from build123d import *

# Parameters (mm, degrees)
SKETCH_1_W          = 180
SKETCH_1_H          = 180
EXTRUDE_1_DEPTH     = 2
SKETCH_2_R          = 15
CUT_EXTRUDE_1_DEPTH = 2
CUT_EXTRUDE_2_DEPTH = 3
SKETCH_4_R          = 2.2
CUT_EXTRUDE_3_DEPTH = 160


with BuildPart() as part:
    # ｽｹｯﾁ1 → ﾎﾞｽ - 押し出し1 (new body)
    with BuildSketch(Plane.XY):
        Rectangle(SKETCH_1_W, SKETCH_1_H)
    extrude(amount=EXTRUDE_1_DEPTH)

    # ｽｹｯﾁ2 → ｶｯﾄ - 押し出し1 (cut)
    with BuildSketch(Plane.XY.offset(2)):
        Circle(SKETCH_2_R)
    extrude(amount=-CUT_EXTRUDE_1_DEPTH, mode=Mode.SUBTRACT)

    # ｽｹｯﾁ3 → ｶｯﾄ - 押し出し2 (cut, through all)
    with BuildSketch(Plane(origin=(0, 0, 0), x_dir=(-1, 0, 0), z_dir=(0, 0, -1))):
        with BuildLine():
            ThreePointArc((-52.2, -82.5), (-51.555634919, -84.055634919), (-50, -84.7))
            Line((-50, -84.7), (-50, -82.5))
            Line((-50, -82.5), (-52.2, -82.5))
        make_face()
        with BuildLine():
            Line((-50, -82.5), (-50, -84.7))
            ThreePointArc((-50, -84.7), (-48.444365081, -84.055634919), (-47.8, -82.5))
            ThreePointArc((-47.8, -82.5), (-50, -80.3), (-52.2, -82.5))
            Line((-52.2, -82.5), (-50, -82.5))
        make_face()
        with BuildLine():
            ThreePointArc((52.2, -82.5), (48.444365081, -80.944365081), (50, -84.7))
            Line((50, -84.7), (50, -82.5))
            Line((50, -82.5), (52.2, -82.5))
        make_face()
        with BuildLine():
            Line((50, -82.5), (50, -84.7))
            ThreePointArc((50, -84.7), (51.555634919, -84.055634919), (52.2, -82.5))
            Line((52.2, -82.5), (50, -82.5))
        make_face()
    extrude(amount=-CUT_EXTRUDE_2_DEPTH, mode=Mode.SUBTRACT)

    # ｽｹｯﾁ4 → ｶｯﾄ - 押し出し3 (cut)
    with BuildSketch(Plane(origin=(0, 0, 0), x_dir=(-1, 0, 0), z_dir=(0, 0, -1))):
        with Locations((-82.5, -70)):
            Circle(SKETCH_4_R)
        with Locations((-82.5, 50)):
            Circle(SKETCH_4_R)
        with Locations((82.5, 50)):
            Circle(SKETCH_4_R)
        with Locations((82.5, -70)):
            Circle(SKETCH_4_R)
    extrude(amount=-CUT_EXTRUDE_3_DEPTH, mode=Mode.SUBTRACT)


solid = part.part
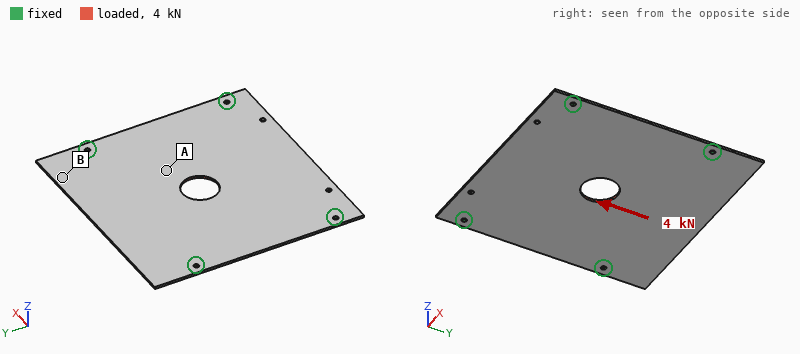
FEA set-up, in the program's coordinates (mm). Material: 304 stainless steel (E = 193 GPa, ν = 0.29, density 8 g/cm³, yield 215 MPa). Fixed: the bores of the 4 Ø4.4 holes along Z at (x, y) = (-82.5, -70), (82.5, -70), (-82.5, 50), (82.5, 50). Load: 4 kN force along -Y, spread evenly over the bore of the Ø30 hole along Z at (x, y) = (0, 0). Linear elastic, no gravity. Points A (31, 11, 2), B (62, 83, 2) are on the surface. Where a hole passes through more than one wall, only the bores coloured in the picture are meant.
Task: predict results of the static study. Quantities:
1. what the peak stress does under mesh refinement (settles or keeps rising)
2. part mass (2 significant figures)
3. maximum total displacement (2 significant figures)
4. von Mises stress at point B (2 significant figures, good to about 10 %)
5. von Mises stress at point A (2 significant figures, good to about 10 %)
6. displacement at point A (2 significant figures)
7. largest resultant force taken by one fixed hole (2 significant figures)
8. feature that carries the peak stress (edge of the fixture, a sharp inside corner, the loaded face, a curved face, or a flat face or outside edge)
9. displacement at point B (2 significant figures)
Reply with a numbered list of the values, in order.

1. keeps rising
2. 510 g
3. 11 µm
4. 5.5 MPa
5. 14 MPa
6. 7.7 µm
7. 1.1 kN
8. edge of the fixture
9. 5.0 µm
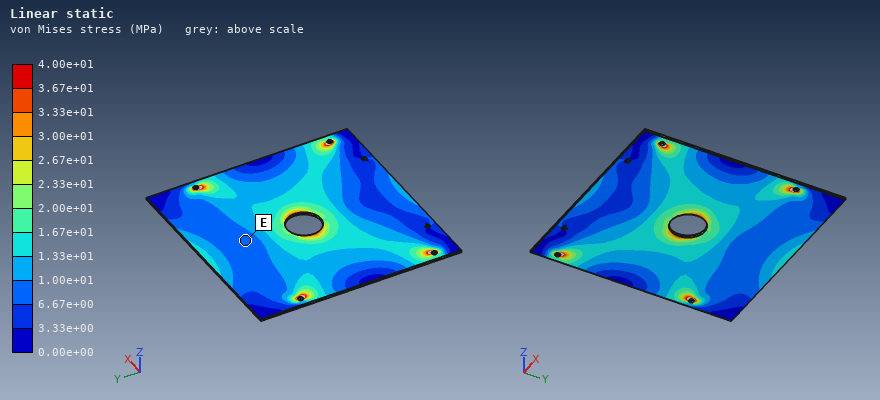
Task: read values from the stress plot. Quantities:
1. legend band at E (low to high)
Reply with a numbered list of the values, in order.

1. 6.67e+00 to 1.00e+01 MPa
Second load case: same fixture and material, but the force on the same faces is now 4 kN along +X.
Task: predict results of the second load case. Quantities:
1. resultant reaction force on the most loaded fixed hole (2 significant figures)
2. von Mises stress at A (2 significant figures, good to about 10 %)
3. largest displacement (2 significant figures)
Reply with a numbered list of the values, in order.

1. 1.2 kN
2. 15 MPa
3. 8.8 µm
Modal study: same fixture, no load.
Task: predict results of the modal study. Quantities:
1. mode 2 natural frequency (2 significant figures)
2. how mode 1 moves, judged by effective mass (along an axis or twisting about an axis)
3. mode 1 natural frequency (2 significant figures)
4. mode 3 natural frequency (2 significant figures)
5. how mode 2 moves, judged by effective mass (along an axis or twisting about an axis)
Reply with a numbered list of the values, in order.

1. 360 Hz
2. along Z
3. 290 Hz
4. 510 Hz
5. twisting about X
